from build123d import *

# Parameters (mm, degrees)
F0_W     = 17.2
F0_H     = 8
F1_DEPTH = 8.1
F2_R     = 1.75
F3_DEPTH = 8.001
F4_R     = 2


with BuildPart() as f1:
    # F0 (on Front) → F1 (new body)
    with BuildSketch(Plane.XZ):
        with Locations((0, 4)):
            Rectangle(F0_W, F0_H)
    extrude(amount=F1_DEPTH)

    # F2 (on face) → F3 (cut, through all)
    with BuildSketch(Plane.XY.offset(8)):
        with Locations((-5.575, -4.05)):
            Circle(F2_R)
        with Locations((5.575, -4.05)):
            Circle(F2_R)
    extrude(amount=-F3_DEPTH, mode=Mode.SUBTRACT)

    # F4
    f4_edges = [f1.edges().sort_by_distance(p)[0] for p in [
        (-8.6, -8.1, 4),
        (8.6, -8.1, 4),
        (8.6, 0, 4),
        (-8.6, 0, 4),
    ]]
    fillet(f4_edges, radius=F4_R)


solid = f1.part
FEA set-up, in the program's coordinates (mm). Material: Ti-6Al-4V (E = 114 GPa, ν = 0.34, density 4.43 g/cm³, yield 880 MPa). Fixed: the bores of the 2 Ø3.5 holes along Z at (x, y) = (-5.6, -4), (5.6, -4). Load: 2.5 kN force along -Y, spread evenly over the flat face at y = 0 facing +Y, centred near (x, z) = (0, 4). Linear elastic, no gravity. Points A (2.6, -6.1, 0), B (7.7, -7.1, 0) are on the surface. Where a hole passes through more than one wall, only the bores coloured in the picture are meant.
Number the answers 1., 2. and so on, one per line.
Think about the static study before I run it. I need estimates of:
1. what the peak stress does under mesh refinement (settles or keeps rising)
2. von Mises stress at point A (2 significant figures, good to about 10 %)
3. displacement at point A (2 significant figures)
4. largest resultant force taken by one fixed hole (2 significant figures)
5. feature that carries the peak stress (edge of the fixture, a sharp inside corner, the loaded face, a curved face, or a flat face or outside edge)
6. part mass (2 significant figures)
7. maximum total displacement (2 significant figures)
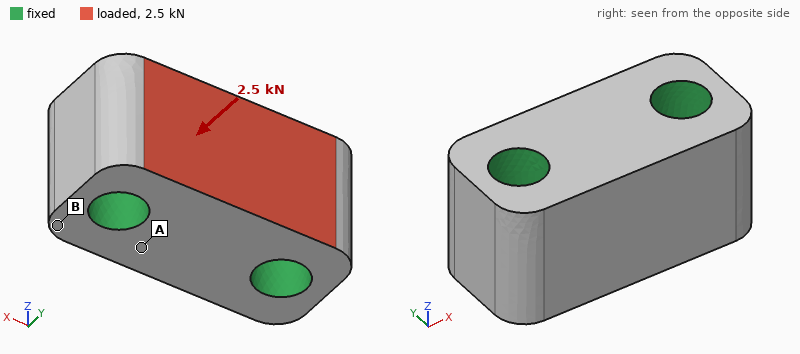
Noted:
1. keeps rising
2. 17 MPa
3. 0.53 µm
4. 1.3 kN
5. edge of the fixture
6. 4.1 g
7. 1.7 µm
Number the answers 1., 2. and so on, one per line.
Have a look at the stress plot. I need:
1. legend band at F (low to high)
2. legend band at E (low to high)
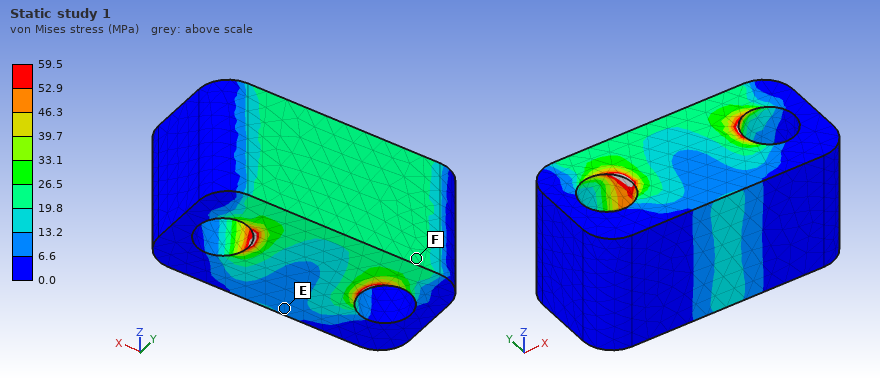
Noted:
1. 19.8 to 26.5 MPa
2. 6.6 to 13.2 MPa
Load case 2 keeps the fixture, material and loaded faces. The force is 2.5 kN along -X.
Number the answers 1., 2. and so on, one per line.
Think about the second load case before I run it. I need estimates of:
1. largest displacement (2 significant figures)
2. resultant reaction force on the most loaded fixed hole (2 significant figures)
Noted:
1. 1.7 µm
2. 1.4 kN
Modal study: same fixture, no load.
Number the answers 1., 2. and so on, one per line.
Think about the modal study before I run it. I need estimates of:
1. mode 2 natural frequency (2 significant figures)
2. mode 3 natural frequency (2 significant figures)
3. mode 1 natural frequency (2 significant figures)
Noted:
1. 150 kHz
2. 150 kHz
3. 140 kHz
